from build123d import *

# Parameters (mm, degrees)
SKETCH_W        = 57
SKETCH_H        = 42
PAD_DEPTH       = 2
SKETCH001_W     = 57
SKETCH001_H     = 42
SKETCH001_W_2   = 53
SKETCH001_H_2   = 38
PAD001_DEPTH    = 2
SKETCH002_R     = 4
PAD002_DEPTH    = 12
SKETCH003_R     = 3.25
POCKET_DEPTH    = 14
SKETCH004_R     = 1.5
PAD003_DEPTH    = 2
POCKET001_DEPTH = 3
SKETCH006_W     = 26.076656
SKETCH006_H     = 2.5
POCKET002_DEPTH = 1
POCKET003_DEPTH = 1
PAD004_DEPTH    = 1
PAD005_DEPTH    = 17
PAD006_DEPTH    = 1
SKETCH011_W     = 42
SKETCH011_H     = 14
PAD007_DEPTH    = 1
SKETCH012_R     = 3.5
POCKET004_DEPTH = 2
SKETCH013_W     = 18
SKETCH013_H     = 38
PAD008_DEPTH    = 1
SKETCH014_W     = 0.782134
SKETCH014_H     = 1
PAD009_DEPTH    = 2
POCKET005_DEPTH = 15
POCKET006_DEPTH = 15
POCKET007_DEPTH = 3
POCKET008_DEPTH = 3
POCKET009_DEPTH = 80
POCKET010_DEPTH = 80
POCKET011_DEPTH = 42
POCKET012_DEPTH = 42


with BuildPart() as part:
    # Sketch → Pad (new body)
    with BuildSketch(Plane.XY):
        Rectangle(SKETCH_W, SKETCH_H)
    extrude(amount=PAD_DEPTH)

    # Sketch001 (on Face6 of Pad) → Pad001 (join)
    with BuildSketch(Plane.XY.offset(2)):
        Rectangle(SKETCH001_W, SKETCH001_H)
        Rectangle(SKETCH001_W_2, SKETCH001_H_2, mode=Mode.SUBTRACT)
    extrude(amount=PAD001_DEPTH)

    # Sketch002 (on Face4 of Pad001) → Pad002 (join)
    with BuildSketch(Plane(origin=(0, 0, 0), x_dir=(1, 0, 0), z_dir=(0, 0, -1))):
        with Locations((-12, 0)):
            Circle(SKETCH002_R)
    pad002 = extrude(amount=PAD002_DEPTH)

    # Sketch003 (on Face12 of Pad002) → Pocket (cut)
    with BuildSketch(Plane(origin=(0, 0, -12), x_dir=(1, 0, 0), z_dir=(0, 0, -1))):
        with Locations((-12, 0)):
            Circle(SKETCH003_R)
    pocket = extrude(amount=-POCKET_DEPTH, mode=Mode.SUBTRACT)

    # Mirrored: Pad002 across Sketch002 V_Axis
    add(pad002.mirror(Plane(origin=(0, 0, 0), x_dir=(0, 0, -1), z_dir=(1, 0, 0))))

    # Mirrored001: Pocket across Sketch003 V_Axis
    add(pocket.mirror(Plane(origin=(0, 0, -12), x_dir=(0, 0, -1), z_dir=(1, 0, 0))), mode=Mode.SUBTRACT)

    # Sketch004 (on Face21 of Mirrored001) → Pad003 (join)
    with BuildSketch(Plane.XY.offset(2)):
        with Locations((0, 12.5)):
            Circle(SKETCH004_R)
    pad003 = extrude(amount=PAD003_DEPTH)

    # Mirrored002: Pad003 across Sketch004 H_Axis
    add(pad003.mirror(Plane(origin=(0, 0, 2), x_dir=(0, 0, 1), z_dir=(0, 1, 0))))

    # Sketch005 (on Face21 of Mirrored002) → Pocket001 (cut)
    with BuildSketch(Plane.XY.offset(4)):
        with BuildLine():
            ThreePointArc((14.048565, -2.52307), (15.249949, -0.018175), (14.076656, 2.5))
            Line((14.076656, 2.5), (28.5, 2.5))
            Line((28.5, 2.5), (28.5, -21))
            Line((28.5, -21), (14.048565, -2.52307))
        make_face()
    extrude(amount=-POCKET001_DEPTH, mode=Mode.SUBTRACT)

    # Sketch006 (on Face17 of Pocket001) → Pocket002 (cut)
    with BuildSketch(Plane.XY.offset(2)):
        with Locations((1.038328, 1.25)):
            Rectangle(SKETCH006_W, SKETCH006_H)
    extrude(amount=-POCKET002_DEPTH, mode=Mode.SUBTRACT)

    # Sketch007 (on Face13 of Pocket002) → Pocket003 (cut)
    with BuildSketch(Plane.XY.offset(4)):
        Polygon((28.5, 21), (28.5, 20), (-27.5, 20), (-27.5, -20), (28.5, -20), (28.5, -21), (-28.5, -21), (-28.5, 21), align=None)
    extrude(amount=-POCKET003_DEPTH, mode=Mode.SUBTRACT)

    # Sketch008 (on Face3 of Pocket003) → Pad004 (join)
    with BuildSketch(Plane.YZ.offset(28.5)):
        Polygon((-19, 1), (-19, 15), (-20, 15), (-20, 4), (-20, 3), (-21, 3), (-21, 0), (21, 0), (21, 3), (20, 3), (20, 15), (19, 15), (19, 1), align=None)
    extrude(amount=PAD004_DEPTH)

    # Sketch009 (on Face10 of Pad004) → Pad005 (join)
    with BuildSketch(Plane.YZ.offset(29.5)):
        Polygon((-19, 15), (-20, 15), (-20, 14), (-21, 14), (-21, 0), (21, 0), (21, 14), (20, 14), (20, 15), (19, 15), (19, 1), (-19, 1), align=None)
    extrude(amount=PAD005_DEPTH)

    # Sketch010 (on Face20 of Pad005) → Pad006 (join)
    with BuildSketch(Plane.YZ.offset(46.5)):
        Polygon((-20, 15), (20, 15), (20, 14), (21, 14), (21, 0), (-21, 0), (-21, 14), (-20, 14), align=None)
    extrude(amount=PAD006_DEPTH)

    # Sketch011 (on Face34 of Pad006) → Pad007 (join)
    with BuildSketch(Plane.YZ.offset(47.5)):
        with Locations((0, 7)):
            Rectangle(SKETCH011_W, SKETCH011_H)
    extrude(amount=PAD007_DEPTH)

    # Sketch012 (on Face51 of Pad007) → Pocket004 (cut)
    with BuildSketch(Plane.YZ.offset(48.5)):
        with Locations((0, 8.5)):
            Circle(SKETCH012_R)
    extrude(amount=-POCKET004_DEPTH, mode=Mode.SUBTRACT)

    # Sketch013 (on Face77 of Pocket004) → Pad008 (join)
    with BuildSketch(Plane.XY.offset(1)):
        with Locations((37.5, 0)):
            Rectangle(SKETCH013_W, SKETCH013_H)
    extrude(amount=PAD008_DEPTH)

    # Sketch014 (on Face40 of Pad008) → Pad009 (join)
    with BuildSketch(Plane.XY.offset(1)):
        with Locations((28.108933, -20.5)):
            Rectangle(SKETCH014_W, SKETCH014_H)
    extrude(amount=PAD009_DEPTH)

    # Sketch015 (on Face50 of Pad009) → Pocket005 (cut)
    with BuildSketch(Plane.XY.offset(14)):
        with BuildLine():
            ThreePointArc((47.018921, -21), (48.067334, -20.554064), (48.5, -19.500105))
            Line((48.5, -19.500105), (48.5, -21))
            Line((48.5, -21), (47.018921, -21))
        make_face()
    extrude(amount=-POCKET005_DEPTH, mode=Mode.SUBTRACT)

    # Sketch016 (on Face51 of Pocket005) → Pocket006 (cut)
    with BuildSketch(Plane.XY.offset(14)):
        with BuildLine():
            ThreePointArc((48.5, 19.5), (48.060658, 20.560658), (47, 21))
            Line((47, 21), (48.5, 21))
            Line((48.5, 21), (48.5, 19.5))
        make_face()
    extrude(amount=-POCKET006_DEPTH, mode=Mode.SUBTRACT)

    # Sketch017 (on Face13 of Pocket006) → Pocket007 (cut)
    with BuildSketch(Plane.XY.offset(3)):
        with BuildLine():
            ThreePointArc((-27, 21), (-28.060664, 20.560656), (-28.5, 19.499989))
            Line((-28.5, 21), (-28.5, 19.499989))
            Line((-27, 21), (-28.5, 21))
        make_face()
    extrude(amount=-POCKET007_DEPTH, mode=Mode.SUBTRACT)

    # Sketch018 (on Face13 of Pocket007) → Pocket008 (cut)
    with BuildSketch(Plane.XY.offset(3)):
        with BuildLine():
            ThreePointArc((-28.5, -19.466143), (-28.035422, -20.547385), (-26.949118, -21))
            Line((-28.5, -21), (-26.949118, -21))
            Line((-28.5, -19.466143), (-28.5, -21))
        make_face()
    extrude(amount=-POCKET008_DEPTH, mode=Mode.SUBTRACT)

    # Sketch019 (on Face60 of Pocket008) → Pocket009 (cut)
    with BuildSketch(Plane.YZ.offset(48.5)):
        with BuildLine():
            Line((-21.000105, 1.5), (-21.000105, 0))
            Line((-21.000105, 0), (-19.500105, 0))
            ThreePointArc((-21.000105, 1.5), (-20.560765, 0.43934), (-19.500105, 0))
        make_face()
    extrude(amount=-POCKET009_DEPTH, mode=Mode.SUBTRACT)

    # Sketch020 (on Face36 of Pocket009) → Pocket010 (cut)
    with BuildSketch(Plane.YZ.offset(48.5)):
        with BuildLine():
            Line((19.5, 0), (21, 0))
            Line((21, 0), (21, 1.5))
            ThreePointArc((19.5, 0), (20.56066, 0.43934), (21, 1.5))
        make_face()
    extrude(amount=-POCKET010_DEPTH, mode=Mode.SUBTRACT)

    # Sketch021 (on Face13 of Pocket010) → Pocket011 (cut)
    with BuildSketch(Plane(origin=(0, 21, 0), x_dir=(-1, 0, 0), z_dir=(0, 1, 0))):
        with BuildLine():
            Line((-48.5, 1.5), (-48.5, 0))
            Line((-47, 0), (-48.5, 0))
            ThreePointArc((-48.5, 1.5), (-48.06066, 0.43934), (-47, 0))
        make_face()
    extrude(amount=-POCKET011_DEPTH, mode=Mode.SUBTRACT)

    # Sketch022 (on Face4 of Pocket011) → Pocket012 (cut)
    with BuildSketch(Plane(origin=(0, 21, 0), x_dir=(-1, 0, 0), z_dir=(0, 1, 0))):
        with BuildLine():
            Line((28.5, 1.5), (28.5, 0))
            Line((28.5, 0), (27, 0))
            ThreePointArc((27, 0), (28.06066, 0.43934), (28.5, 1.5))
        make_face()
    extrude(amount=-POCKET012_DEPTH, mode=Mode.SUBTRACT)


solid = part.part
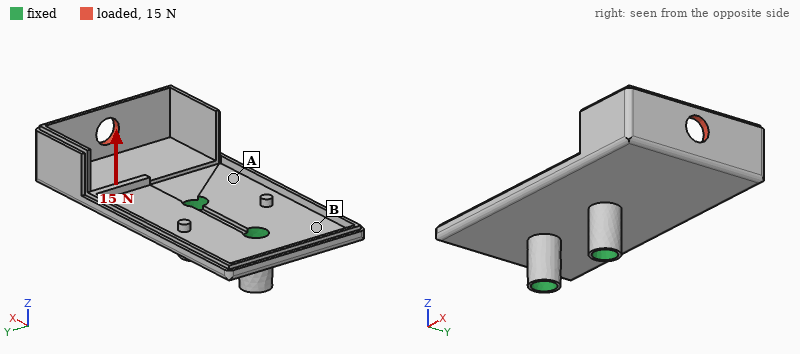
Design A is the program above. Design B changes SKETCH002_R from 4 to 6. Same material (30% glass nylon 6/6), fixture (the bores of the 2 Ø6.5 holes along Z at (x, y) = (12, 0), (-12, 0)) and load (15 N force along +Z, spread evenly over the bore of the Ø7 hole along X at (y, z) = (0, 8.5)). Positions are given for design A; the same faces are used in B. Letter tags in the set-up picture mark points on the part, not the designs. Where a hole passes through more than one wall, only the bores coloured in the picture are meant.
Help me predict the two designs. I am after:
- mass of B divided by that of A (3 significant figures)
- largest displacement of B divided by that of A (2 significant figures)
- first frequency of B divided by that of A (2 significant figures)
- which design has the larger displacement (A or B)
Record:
1.17
0.86
1.1
A
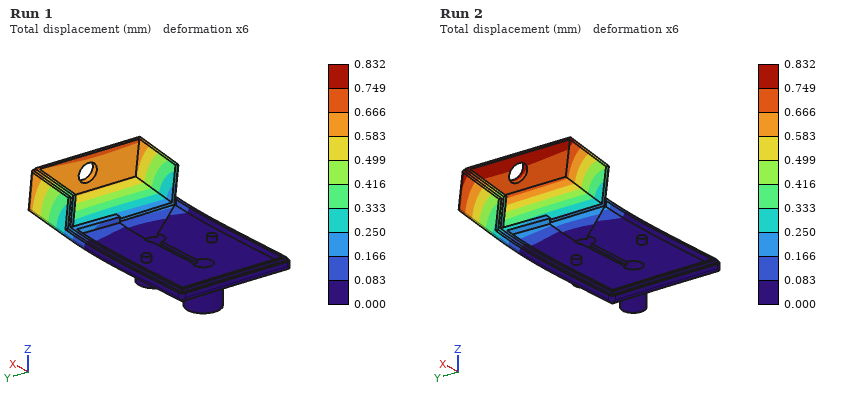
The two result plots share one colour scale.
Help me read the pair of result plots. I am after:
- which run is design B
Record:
Run 1
